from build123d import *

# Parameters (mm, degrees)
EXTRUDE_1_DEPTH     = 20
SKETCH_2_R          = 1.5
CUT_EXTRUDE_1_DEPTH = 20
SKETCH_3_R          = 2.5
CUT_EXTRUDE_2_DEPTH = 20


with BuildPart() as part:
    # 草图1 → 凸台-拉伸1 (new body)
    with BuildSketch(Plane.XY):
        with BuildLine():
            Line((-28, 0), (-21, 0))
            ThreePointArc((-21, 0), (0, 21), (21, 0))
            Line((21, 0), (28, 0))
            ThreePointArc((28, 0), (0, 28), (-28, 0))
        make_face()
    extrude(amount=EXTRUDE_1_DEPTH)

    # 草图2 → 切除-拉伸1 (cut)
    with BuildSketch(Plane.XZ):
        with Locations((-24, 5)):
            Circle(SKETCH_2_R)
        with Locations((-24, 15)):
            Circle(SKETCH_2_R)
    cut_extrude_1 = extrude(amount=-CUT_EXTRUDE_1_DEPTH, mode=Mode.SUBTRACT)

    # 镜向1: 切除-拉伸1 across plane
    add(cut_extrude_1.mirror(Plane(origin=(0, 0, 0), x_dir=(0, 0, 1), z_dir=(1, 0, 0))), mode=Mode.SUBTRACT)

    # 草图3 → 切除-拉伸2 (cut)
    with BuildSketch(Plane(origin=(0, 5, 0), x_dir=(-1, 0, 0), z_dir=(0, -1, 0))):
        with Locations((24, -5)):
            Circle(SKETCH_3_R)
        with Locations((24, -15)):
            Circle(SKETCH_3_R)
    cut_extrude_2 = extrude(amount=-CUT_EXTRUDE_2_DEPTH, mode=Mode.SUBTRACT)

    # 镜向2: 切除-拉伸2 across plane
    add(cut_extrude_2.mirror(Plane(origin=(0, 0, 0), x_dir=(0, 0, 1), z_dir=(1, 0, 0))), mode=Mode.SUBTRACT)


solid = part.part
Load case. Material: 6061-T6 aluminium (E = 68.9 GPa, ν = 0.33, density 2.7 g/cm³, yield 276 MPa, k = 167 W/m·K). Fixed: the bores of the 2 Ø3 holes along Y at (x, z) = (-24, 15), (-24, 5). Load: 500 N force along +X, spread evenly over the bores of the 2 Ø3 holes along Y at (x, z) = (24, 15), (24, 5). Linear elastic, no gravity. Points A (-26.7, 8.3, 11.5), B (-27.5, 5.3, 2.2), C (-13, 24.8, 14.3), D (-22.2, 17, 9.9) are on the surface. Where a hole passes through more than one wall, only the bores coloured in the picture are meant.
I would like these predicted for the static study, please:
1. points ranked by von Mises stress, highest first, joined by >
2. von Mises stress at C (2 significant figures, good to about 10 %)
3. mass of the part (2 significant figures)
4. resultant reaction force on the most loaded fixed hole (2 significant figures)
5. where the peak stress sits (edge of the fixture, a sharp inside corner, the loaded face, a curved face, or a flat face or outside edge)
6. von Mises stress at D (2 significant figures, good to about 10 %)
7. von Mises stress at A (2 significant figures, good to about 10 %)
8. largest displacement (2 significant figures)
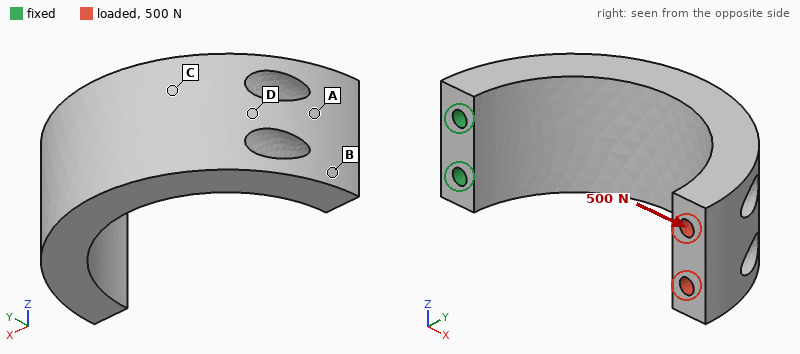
C > D > A > B
48 MPa
27 g
250 N
a curved face
37 MPa
17 MPa
0.46 mm
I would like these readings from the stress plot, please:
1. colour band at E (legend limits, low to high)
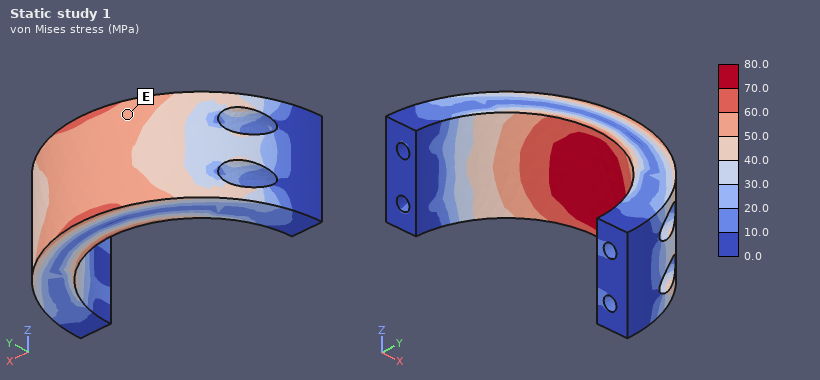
50.0 to 60.0 MPa
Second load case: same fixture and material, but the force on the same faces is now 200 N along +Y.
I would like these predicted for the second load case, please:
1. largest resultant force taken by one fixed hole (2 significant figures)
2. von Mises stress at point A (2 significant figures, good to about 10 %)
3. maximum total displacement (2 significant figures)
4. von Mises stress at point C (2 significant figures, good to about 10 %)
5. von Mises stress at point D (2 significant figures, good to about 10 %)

140 N
65 MPa
0.46 mm
37 MPa
57 MPa
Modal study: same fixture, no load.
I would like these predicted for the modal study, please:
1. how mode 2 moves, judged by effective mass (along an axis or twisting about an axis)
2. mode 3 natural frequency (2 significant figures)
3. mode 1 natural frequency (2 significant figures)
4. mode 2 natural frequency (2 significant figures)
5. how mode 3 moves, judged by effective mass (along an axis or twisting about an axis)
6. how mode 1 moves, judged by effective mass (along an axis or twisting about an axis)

along Z
3700 Hz
1200 Hz
1600 Hz
along X
along Y
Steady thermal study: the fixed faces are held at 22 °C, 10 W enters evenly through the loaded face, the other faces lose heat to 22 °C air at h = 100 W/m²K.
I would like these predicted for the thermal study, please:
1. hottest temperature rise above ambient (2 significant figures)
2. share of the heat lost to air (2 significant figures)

23 K
49 %
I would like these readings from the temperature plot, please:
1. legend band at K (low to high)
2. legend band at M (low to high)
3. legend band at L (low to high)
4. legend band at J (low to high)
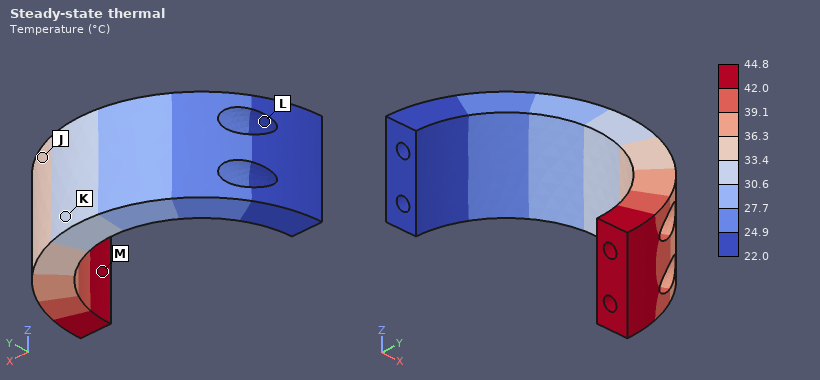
30.6 to 33.4 °C
42.0 to 44.8 °C
22.0 to 24.9 °C
33.4 to 36.3 °C
